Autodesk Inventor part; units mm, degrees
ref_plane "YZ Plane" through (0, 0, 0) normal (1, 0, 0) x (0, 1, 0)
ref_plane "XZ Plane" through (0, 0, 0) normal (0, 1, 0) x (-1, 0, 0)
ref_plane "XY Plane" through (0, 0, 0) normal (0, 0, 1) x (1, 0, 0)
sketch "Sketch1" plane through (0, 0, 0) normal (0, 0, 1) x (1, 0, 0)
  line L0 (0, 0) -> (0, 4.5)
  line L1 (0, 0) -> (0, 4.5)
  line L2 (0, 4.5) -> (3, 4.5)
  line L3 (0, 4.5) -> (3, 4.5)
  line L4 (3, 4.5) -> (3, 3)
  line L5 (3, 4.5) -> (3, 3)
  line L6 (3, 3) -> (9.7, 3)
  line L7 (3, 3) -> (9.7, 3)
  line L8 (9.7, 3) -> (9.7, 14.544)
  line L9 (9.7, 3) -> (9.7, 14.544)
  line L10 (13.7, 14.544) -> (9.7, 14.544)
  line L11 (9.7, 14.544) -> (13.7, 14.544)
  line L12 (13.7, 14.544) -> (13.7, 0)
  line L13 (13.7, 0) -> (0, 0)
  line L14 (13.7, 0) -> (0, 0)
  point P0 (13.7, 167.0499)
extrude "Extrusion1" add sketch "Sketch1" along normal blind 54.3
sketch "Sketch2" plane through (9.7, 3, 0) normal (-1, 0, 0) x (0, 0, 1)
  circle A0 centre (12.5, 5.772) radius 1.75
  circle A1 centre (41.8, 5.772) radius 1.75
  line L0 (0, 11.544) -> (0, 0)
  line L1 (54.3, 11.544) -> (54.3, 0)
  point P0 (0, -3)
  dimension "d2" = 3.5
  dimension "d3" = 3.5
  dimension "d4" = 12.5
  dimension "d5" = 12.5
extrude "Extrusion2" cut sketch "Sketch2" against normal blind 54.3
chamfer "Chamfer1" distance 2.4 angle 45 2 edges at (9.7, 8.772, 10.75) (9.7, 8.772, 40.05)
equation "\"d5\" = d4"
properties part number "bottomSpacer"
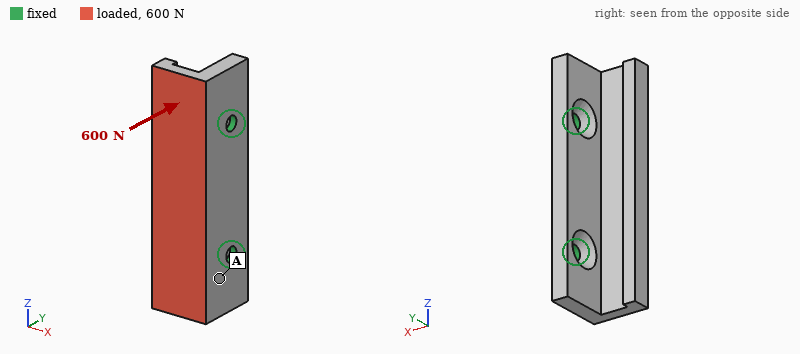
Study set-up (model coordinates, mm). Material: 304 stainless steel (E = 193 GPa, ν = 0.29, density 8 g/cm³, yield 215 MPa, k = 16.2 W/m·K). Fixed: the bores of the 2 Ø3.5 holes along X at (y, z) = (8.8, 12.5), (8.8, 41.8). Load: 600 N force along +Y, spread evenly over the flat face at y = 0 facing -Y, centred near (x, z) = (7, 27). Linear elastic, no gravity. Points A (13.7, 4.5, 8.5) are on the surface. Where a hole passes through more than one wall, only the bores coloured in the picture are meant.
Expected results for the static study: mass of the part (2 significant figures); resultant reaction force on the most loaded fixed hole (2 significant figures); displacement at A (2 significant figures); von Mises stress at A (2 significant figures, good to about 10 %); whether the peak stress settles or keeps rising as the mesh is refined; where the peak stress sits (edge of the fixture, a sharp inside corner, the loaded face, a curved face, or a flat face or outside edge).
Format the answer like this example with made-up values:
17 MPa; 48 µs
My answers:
39 g; 300 N; 3.6 µm; 24 MPa; keeps rising; edge of the fixture
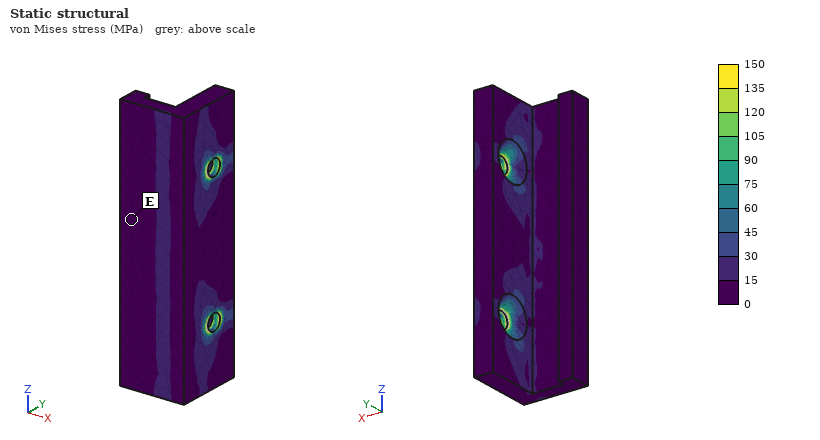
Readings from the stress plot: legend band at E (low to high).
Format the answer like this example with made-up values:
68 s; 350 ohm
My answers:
0 to 15 MPa
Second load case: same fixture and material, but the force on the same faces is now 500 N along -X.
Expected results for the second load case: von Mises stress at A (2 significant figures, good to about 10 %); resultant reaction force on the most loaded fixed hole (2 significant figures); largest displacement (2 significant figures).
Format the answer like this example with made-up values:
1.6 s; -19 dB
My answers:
23 MPa; 250 N; 20 µm
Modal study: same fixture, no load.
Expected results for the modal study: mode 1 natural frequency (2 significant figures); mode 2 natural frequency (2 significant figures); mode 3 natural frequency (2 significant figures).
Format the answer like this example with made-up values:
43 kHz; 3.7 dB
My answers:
5900 Hz; 8400 Hz; 16 kHz
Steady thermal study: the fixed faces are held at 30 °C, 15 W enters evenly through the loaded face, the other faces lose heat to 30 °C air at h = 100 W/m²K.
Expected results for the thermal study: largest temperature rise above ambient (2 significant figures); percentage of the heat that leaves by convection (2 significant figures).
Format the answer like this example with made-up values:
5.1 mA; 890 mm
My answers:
50 K; 51 %
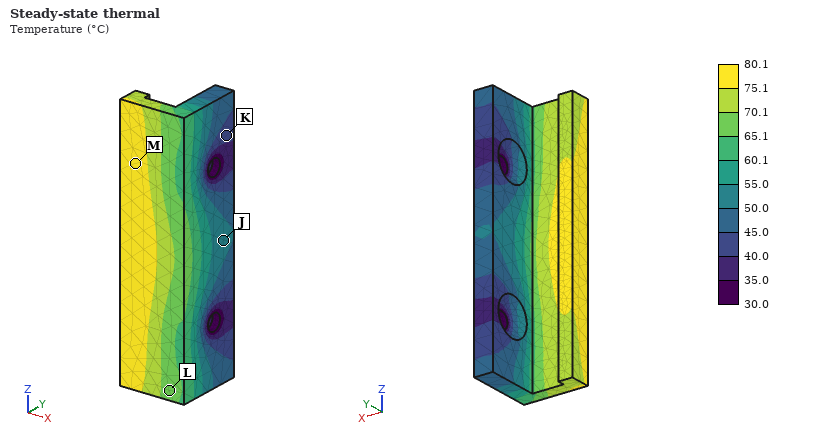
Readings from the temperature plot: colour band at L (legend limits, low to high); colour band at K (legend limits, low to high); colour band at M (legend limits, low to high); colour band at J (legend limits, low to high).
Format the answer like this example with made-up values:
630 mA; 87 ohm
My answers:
65.1 to 70.1 °C; 40.0 to 45.0 °C; 75.1 to 80.1 °C; 50.0 to 55.0 °C
